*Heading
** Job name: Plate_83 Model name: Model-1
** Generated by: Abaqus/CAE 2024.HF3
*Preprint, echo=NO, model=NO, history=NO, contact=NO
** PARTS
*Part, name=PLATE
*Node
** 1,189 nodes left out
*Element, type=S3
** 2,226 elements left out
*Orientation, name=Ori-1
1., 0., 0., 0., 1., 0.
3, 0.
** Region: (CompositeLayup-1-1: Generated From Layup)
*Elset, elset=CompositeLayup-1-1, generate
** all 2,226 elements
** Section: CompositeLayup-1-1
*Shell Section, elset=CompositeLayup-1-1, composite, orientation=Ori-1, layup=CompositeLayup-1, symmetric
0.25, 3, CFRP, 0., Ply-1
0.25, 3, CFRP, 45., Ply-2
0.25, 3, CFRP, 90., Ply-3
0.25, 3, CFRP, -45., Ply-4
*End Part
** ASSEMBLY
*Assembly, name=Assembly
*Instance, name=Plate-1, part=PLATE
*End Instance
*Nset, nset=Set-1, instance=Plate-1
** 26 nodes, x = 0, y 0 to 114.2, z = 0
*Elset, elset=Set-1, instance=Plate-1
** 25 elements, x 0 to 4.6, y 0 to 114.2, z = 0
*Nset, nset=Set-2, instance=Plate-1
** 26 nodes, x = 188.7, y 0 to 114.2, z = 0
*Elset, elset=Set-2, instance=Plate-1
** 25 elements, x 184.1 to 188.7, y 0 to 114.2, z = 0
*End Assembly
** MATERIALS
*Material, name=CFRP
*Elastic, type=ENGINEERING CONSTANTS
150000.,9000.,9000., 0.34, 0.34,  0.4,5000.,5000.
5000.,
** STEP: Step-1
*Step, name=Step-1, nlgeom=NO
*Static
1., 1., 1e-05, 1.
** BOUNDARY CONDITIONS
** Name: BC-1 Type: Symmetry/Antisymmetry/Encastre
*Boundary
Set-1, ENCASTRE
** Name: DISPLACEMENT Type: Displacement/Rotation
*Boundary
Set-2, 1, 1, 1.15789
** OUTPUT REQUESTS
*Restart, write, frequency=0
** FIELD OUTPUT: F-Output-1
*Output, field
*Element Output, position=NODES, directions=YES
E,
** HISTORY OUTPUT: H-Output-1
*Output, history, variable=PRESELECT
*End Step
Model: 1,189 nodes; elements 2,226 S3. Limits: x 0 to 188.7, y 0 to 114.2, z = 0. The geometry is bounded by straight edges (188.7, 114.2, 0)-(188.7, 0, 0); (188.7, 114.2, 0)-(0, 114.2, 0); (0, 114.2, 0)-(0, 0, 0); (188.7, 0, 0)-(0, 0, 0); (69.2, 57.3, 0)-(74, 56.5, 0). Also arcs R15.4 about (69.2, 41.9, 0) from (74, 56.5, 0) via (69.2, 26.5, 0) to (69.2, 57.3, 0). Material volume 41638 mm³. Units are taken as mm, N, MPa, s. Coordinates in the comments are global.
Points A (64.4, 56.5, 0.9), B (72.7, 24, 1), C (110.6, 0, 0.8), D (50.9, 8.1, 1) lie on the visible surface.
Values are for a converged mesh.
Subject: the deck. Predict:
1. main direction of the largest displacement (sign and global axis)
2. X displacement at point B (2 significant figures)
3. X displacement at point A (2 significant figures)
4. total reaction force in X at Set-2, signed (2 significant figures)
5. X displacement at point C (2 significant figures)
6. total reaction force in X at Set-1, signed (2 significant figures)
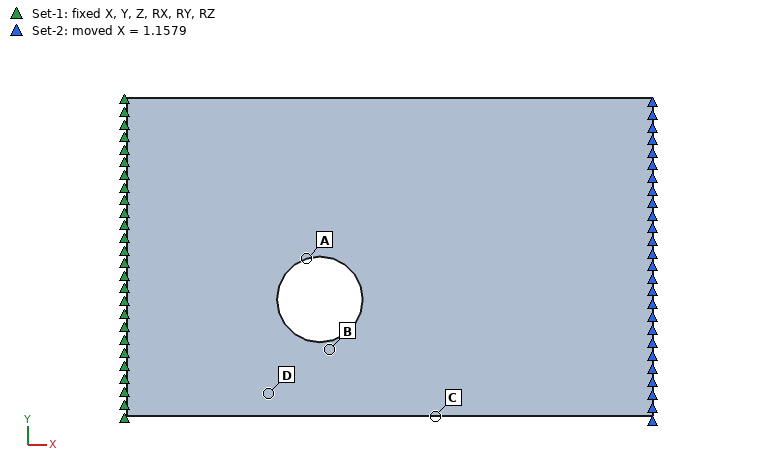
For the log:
+X
0.49 mm
0.35 mm
72000 N
0.72 mm
-72000 N
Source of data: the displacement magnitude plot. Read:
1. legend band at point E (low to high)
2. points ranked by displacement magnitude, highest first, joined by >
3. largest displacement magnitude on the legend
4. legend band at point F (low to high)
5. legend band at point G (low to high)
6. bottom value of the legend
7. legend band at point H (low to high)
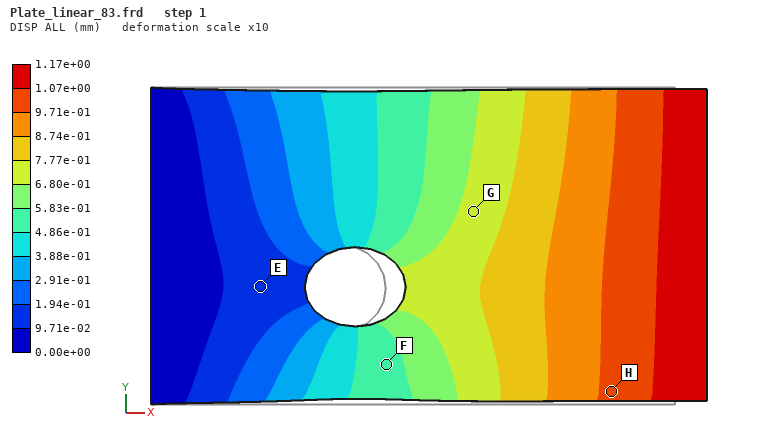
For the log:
9.71e-02 to 1.94e-01 mm
H > G > F > E
1.17e+00 mm
4.86e-01 to 5.83e-01 mm
6.80e-01 to 7.77e-01 mm
0.00e+00 mm
9.71e-01 to 1.07e+00 mm
